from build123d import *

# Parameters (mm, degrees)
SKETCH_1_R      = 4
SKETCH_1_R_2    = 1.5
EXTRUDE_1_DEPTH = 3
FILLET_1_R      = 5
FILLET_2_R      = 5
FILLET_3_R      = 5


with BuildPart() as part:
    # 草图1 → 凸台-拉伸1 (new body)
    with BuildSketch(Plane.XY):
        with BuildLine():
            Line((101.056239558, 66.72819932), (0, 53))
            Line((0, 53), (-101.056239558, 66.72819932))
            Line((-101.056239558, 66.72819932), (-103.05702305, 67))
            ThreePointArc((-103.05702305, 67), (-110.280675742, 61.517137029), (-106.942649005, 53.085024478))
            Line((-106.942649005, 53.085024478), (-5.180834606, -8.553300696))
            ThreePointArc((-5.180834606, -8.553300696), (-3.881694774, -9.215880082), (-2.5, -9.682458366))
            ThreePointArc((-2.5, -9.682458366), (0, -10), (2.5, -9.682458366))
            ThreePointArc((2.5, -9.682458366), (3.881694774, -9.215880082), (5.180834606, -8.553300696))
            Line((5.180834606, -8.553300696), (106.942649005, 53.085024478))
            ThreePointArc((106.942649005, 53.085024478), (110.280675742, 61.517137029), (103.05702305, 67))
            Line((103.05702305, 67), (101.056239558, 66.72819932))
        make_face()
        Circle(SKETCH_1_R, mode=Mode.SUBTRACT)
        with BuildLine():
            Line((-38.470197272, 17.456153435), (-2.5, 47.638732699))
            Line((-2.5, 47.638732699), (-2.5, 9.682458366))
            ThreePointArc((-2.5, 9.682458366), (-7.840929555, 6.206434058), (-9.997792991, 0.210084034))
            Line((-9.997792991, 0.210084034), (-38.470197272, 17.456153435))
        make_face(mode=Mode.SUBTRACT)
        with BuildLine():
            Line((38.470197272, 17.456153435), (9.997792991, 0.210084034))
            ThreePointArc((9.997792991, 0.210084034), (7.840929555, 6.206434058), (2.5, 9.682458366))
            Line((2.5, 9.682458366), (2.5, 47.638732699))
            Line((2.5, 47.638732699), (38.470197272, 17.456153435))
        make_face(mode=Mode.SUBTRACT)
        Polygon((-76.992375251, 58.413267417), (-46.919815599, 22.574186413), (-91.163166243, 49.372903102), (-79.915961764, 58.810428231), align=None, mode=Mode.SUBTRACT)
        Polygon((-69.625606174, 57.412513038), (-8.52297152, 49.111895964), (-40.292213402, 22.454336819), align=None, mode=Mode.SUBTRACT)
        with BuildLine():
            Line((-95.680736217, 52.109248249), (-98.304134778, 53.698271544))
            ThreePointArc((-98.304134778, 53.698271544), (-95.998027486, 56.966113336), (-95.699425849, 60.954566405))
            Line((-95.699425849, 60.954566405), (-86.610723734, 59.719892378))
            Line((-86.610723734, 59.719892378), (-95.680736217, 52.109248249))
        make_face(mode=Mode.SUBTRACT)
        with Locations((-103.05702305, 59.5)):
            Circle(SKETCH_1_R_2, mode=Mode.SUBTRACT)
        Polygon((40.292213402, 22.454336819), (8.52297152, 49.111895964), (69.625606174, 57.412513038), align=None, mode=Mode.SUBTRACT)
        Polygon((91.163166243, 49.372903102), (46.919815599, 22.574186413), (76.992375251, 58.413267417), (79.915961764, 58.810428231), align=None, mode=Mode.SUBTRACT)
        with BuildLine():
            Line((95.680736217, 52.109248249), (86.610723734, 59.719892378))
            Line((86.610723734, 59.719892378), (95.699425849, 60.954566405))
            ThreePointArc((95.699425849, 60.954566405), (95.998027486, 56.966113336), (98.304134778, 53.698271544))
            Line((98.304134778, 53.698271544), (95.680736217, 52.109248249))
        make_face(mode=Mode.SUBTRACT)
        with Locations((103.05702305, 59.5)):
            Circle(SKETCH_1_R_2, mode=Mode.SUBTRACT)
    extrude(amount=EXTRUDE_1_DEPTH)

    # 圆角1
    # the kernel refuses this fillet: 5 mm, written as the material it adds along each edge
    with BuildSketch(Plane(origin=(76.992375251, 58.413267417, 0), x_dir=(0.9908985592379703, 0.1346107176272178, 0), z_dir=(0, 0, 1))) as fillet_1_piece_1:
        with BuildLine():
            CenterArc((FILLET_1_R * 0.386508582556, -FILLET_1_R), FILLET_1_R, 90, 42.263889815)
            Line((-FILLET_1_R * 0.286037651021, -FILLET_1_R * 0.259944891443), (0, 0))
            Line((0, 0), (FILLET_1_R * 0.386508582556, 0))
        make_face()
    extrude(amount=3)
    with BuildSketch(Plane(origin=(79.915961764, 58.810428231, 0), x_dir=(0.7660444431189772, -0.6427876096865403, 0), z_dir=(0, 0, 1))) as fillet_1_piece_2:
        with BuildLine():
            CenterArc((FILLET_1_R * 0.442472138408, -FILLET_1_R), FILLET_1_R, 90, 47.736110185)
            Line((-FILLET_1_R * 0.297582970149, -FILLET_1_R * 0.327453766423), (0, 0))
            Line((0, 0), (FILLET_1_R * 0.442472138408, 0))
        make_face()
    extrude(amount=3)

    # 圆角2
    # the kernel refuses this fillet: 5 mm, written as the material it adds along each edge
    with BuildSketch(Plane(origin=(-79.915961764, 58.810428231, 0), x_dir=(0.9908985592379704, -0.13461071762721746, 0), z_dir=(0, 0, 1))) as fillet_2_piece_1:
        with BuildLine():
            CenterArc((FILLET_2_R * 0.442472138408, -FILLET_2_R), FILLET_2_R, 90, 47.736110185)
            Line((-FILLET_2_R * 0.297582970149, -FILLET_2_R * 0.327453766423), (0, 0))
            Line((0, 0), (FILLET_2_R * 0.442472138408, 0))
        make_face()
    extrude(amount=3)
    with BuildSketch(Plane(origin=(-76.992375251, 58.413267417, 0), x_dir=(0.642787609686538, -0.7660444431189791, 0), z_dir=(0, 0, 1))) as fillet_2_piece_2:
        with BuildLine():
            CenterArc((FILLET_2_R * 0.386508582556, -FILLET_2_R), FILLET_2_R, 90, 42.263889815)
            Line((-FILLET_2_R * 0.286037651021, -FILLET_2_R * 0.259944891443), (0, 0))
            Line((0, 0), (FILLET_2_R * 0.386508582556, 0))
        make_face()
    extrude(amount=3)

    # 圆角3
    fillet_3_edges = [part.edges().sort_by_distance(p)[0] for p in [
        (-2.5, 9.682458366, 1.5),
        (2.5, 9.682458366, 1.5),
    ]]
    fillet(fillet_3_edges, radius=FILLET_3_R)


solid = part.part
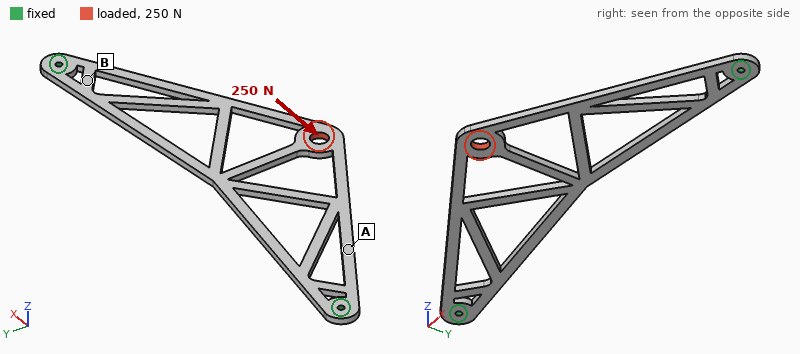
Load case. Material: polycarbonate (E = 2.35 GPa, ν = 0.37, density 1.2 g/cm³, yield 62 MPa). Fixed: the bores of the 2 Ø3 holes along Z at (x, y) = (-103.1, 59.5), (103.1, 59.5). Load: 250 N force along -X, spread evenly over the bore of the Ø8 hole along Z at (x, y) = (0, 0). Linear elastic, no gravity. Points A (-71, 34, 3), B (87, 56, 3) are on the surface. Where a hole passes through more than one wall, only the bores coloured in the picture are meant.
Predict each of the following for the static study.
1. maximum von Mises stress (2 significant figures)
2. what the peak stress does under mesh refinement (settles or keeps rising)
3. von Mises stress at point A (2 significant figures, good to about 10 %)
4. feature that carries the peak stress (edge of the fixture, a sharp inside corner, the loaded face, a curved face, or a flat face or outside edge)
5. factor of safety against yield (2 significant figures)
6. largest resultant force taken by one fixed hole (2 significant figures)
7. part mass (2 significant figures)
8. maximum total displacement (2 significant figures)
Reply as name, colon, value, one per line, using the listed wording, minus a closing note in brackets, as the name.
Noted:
maximum von Mises stress: 43 MPa
what the peak stress does under mesh refinement: settles
von Mises stress at point A: 6.8 MPa
feature that carries the peak stress: a flat face or outside edge
factor of safety against yield: 1.4
largest resultant force taken by one fixed hole: 140 N
part mass: 14 g
maximum total displacement: 1.3 mm
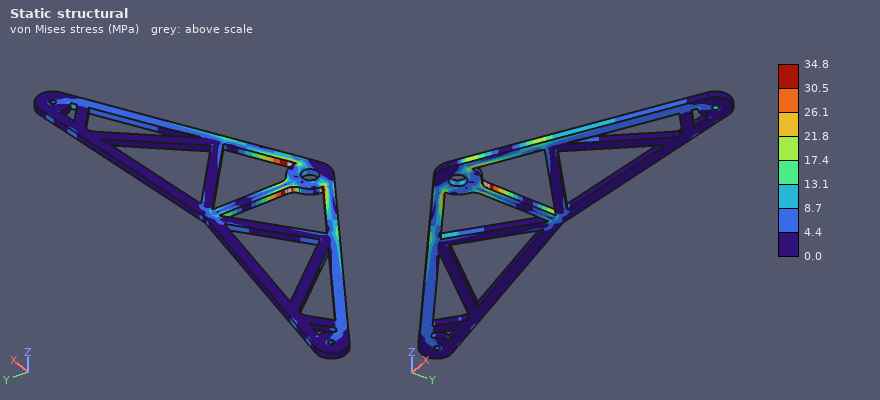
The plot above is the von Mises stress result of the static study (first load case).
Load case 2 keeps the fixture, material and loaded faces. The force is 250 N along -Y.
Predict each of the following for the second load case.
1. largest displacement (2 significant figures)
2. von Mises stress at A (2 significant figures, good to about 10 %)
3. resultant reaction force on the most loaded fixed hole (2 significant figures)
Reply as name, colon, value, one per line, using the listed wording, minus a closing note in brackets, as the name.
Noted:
largest displacement: 1.1 mm
von Mises stress at A: 9.8 MPa
resultant reaction force on the most loaded fixed hole: 220 N
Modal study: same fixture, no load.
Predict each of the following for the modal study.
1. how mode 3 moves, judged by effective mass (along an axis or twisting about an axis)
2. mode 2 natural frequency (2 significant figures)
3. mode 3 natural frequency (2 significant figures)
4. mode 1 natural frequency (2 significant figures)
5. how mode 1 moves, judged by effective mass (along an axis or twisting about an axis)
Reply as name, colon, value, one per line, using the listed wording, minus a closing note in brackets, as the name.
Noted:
how mode 3 moves, judged by effective mass: twisting about Y
mode 2 natural frequency: 150 Hz
mode 3 natural frequency: 200 Hz
mode 1 natural frequency: 61 Hz
how mode 1 moves, judged by effective mass: along Z
